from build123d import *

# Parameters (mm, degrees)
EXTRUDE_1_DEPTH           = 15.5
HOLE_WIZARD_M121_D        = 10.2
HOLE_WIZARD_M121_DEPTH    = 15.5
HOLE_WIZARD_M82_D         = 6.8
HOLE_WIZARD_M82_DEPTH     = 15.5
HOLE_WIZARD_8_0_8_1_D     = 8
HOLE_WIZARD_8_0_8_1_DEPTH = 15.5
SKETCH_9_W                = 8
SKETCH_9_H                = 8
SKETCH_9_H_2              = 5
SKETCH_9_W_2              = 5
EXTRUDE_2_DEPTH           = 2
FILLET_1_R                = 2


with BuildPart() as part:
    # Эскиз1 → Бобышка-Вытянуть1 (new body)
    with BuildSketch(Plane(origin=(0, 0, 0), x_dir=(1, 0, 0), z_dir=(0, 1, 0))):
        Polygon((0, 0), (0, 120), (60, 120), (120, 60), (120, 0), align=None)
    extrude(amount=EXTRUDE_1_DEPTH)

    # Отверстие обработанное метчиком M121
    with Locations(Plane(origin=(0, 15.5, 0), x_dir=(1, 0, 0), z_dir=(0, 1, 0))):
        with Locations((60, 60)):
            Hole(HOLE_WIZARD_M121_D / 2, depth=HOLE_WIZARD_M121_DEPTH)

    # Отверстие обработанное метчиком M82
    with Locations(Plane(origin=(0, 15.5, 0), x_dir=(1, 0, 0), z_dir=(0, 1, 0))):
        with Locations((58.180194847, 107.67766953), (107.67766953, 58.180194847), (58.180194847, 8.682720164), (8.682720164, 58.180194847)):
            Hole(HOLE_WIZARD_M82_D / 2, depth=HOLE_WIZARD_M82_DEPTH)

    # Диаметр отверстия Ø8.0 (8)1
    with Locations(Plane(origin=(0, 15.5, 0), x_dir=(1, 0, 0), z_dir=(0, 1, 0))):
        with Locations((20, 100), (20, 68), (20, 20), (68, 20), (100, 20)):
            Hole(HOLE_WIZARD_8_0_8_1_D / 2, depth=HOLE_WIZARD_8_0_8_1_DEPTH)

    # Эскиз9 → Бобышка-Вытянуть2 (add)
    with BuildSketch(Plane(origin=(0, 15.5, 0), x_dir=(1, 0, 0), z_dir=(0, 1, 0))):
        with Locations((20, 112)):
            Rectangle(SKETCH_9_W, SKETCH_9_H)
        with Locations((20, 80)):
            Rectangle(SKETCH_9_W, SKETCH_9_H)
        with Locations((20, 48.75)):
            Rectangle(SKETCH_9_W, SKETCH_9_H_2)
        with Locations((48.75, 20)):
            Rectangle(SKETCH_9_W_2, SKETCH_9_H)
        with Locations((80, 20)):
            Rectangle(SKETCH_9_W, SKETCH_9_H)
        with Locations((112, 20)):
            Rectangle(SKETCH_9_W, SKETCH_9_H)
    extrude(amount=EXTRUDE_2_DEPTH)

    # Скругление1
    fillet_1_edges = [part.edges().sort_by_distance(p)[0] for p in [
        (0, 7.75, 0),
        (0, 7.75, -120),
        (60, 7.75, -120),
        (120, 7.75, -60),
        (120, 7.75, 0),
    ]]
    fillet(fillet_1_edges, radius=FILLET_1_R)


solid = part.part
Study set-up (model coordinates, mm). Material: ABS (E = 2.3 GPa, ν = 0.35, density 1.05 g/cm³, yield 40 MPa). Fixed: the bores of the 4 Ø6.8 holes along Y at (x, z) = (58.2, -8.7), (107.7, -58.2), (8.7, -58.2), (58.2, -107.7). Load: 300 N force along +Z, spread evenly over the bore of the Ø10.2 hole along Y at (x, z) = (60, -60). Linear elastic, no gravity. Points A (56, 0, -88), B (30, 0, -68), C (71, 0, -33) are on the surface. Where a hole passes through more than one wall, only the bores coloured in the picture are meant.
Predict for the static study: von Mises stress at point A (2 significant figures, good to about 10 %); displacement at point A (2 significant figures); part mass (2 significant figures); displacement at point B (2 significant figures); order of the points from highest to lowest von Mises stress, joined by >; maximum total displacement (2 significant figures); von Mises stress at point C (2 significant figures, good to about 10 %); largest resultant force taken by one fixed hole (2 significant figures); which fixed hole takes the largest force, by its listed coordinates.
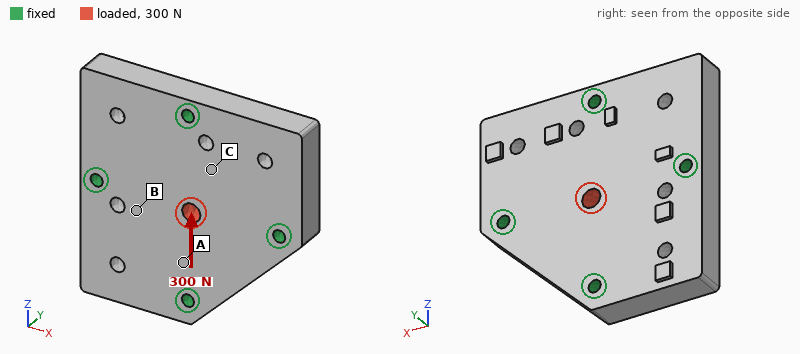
0.33 MPa
2.6 µm
200 g
2.0 µm
A > C > B
7.0 µm
0.17 MPa
110 N
(58.2, -107.7)
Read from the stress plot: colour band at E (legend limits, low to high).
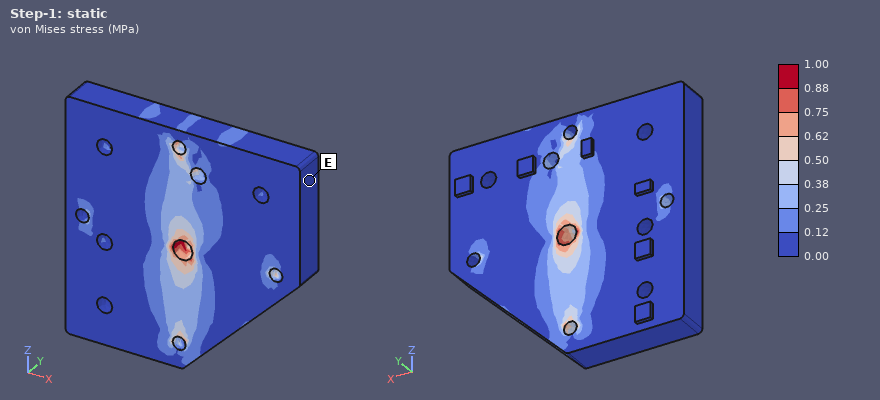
0.00 to 0.12 MPa
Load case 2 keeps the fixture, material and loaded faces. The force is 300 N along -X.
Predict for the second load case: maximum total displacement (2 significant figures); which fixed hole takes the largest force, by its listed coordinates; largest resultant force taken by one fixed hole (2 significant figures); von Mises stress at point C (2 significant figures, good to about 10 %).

7.1 µm
(107.7, -58.2)
110 N
0.074 MPa
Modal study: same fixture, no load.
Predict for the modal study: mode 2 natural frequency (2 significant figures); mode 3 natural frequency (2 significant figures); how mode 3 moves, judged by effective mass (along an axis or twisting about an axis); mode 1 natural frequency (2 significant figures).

1700 Hz
1900 Hz
along Y
1700 Hz
